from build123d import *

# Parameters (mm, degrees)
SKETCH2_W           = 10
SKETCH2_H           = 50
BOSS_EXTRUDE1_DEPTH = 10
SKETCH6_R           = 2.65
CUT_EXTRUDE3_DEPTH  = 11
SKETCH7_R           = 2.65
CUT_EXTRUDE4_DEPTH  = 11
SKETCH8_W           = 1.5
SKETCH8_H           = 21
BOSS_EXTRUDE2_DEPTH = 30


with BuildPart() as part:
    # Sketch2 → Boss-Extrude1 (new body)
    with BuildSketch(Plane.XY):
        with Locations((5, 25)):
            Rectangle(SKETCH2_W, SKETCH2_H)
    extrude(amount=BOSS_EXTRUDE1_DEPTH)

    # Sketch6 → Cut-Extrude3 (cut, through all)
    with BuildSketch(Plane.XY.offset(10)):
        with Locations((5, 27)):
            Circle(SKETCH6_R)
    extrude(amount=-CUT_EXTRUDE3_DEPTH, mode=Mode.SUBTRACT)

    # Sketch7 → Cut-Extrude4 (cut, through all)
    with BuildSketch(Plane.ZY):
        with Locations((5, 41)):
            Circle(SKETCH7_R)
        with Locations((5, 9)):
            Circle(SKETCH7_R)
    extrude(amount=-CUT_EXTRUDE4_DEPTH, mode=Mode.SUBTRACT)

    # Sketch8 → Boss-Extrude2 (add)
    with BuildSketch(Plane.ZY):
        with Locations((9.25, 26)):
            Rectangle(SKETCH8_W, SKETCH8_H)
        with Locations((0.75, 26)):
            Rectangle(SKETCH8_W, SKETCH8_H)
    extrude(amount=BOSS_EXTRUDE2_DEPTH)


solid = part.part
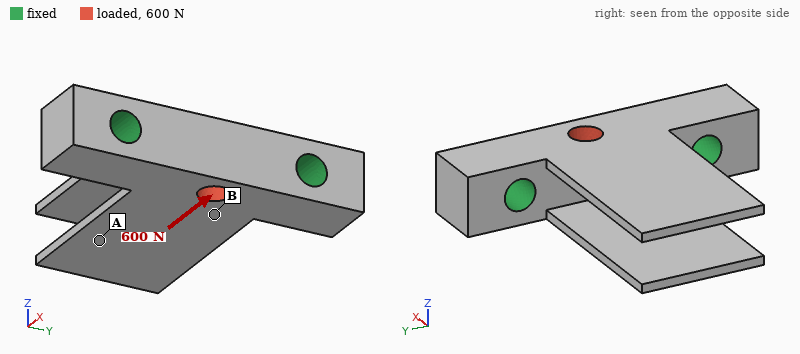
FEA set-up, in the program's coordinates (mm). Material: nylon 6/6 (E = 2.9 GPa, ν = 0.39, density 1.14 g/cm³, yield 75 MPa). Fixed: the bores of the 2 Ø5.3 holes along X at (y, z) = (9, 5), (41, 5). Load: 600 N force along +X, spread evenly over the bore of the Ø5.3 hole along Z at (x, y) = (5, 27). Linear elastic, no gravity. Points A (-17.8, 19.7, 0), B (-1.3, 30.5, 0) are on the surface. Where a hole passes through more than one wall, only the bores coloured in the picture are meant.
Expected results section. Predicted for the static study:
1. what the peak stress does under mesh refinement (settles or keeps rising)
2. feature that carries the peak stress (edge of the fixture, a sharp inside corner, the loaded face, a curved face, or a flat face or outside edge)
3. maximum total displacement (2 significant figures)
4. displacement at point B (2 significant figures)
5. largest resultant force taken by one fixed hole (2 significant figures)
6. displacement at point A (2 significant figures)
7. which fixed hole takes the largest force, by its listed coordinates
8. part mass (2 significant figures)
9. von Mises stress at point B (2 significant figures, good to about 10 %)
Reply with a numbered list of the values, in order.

1. keeps rising
2. edge of the fixture
3. 66 µm
4. 39 µm
5. 350 N
6. 38 µm
7. (41, 5)
8. 7.1 g
9. 5.4 MPa
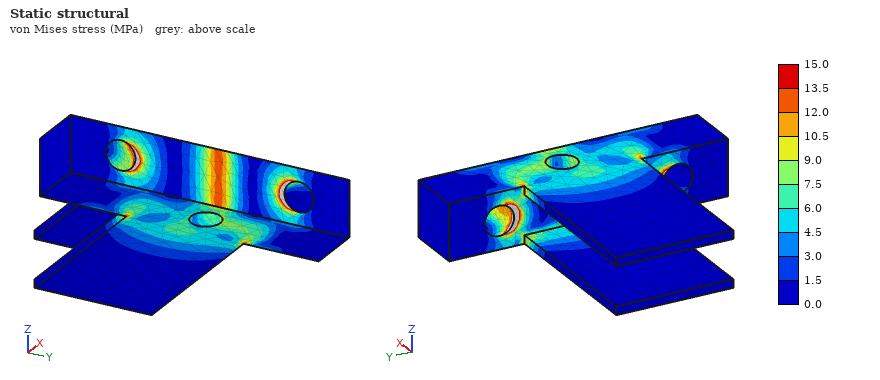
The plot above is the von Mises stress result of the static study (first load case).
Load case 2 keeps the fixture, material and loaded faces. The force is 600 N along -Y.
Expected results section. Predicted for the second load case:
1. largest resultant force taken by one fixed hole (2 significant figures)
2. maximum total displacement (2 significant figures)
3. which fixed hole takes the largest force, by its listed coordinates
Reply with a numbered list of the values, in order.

1. 330 N
2. 16 µm
3. (41, 5)
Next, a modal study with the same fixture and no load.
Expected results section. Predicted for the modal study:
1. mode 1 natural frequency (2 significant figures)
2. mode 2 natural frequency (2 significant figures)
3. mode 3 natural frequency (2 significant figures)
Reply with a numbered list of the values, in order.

1. 420 Hz
2. 420 Hz
3. 1300 Hz
